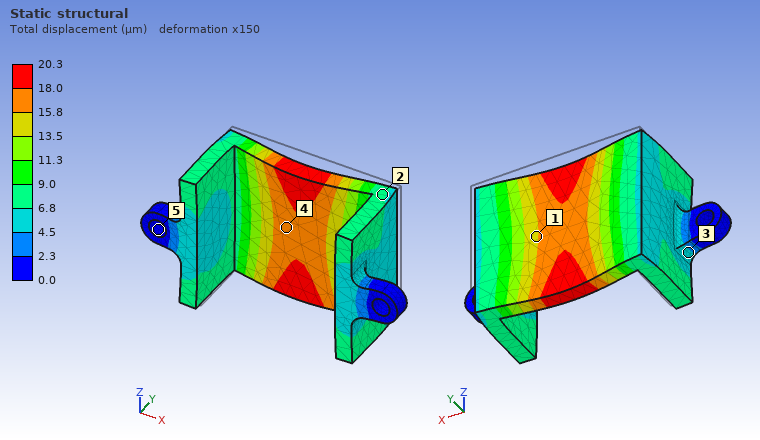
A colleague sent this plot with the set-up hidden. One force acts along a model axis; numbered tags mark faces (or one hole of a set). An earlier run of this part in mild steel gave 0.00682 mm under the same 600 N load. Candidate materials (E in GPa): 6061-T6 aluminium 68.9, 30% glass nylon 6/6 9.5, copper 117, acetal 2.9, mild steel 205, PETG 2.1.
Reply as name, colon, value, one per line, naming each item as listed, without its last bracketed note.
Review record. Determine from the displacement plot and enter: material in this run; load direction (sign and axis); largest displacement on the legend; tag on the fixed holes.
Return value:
material in this run: 6061-T6 aluminium
load direction: -Y
largest displacement on the legend: 20.3 µm
tag on the fixed holes: 5
